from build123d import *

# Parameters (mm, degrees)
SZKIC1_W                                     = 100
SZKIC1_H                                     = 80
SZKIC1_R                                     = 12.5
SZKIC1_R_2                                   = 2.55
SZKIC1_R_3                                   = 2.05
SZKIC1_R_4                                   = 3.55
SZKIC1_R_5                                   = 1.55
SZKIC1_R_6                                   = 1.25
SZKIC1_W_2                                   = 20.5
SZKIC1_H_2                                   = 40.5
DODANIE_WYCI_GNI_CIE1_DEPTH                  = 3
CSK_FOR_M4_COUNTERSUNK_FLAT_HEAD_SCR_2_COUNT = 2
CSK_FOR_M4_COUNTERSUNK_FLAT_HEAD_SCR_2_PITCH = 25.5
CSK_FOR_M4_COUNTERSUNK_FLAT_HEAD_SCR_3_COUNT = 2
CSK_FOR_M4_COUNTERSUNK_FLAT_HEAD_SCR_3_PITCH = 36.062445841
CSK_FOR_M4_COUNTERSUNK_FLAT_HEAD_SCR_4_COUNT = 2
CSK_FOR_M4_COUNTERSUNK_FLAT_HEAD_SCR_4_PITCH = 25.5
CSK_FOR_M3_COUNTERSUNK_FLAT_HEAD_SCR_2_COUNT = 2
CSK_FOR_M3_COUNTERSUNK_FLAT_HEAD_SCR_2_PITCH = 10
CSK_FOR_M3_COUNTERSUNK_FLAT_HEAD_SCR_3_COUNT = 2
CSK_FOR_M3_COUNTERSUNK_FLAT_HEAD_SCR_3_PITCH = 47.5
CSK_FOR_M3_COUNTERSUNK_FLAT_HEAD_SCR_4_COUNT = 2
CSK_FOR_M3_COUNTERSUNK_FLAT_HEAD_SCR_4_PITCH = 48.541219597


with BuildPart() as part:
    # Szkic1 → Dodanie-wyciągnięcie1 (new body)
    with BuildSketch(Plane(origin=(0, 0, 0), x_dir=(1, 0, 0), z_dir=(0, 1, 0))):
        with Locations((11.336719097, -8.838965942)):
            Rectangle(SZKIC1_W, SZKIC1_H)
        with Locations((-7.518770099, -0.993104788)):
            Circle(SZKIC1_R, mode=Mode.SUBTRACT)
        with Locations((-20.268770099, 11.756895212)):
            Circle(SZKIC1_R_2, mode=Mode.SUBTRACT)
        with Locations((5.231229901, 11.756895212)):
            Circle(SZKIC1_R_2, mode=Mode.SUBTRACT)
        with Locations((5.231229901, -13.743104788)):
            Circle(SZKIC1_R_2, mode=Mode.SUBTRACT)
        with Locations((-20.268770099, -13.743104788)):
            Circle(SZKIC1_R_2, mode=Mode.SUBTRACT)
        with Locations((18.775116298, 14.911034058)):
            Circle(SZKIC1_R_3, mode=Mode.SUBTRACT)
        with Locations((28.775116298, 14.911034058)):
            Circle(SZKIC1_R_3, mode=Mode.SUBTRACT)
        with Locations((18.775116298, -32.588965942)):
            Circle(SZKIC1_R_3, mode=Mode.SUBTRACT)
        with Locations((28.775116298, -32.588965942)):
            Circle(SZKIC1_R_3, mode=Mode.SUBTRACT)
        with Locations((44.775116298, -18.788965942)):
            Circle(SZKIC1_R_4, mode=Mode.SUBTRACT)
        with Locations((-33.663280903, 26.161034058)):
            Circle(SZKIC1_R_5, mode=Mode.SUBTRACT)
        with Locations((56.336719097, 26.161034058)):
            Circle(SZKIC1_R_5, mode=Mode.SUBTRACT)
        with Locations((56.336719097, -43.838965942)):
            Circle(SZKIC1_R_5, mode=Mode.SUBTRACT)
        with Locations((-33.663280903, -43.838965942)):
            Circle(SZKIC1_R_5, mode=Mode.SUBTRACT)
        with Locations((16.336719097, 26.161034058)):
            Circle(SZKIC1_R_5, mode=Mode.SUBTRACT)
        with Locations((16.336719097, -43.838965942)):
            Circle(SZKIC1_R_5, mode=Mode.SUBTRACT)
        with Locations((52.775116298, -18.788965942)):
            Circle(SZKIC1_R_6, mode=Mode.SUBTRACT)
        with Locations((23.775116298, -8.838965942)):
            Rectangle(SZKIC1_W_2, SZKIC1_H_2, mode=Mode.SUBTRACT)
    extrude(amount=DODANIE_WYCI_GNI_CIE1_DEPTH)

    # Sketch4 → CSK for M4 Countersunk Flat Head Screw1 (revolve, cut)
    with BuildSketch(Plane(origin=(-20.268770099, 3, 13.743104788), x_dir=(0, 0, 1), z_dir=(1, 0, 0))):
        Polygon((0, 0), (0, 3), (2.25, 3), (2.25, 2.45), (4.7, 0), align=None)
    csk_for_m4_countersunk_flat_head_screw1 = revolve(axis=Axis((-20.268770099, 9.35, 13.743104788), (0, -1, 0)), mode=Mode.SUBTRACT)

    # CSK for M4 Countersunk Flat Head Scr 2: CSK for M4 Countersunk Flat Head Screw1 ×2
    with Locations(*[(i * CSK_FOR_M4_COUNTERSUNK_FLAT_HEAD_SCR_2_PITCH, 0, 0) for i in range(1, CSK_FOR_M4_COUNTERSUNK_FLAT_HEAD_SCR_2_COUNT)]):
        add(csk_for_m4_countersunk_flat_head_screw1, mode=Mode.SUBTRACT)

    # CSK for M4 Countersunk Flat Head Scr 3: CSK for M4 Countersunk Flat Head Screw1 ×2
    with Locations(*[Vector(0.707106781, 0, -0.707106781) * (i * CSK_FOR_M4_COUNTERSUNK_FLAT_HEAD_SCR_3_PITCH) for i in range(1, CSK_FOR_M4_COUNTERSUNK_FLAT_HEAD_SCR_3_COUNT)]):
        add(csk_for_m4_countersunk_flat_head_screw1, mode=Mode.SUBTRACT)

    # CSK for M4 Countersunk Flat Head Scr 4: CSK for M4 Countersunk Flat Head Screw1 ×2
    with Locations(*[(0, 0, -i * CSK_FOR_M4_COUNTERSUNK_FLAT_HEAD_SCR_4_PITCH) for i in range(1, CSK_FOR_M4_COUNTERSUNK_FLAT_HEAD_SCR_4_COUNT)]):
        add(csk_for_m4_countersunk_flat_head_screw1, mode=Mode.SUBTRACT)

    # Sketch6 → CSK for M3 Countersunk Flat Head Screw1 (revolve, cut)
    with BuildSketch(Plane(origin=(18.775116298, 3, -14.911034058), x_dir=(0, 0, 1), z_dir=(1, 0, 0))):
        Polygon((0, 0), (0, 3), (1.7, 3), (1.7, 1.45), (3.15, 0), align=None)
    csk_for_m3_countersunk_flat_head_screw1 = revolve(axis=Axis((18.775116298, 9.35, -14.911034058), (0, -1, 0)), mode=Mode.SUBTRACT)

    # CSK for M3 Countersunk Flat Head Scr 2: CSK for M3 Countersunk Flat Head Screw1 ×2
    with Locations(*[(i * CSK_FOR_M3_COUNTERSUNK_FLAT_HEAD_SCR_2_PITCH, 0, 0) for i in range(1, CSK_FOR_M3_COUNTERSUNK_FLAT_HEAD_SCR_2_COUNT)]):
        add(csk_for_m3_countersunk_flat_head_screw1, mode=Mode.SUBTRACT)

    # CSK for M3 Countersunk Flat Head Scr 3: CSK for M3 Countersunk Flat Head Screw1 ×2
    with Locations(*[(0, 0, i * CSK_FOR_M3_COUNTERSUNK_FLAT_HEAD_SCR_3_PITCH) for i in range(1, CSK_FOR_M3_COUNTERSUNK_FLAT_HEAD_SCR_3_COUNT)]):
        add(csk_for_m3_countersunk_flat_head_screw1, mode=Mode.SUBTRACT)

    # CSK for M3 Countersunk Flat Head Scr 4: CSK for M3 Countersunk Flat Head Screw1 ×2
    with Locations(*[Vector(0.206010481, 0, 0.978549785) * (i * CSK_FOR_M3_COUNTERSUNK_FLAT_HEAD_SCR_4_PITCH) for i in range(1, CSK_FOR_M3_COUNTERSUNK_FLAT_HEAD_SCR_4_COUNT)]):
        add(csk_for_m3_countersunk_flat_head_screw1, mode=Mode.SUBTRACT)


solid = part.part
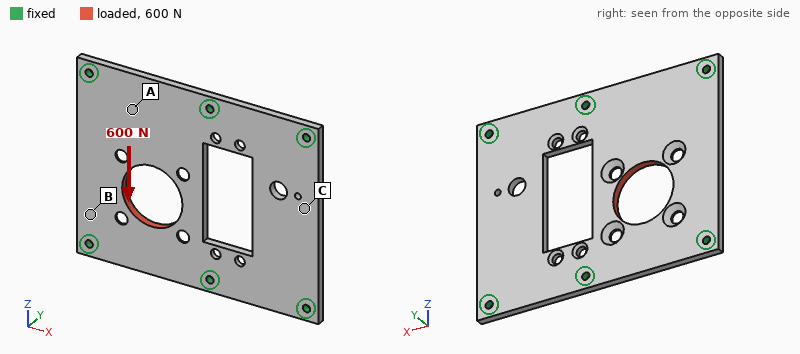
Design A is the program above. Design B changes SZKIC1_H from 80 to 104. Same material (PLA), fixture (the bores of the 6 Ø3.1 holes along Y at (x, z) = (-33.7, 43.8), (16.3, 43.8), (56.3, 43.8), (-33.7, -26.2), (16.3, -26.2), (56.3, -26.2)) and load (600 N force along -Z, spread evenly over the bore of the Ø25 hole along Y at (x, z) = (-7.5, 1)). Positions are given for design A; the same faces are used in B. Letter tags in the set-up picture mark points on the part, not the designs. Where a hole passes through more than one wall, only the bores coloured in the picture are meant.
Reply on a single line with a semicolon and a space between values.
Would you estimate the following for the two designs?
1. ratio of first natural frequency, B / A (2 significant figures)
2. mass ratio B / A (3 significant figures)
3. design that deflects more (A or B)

1.0; 1.38; A
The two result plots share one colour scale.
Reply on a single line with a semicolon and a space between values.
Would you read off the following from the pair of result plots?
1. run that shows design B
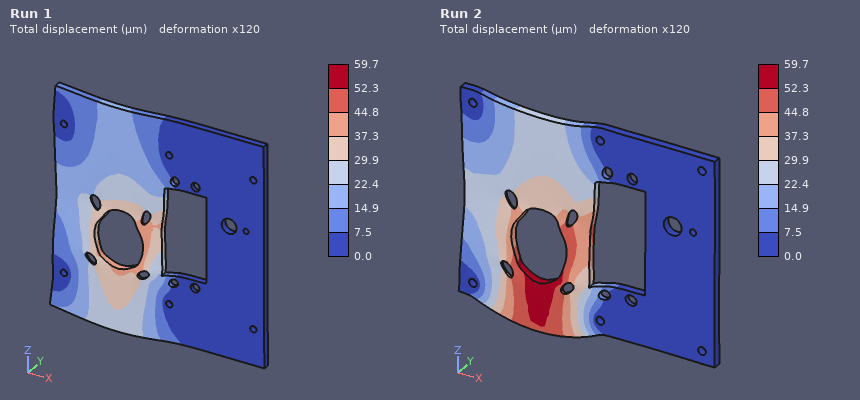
Run 1
